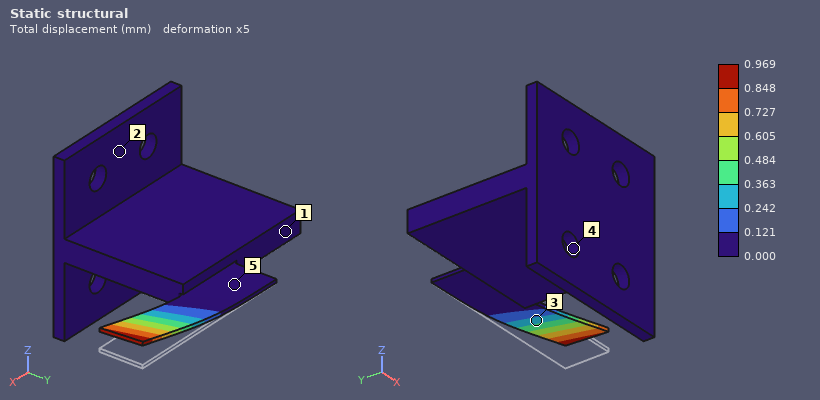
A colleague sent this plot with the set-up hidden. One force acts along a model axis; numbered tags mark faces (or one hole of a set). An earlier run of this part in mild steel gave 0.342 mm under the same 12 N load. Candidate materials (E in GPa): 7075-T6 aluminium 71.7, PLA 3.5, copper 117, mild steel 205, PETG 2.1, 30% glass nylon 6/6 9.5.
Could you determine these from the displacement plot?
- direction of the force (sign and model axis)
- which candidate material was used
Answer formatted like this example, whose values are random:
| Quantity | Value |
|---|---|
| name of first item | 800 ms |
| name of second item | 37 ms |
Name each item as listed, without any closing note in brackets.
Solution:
| Quantity | Value |
|---|---|
| direction of the force | +Z |
| which candidate material was used | 7075-T6 aluminium |
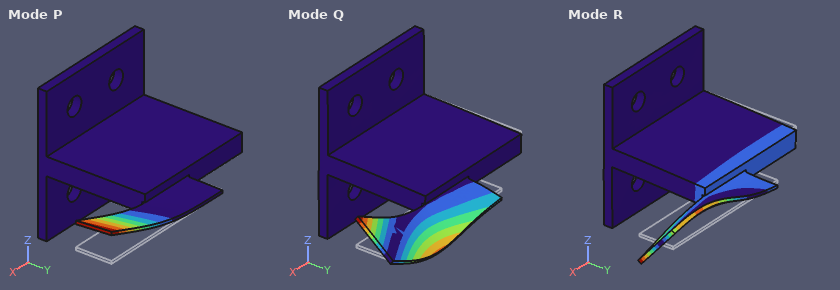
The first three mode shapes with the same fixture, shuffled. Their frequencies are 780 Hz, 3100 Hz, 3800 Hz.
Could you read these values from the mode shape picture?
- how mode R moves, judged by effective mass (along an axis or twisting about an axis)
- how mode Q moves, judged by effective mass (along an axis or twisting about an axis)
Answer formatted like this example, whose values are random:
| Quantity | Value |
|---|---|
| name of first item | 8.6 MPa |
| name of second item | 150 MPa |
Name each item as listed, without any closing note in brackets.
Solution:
| Quantity | Value |
|---|---|
| how mode R moves, judged by effective mass | along Z |
| how mode Q moves, judged by effective mass | along Z |
